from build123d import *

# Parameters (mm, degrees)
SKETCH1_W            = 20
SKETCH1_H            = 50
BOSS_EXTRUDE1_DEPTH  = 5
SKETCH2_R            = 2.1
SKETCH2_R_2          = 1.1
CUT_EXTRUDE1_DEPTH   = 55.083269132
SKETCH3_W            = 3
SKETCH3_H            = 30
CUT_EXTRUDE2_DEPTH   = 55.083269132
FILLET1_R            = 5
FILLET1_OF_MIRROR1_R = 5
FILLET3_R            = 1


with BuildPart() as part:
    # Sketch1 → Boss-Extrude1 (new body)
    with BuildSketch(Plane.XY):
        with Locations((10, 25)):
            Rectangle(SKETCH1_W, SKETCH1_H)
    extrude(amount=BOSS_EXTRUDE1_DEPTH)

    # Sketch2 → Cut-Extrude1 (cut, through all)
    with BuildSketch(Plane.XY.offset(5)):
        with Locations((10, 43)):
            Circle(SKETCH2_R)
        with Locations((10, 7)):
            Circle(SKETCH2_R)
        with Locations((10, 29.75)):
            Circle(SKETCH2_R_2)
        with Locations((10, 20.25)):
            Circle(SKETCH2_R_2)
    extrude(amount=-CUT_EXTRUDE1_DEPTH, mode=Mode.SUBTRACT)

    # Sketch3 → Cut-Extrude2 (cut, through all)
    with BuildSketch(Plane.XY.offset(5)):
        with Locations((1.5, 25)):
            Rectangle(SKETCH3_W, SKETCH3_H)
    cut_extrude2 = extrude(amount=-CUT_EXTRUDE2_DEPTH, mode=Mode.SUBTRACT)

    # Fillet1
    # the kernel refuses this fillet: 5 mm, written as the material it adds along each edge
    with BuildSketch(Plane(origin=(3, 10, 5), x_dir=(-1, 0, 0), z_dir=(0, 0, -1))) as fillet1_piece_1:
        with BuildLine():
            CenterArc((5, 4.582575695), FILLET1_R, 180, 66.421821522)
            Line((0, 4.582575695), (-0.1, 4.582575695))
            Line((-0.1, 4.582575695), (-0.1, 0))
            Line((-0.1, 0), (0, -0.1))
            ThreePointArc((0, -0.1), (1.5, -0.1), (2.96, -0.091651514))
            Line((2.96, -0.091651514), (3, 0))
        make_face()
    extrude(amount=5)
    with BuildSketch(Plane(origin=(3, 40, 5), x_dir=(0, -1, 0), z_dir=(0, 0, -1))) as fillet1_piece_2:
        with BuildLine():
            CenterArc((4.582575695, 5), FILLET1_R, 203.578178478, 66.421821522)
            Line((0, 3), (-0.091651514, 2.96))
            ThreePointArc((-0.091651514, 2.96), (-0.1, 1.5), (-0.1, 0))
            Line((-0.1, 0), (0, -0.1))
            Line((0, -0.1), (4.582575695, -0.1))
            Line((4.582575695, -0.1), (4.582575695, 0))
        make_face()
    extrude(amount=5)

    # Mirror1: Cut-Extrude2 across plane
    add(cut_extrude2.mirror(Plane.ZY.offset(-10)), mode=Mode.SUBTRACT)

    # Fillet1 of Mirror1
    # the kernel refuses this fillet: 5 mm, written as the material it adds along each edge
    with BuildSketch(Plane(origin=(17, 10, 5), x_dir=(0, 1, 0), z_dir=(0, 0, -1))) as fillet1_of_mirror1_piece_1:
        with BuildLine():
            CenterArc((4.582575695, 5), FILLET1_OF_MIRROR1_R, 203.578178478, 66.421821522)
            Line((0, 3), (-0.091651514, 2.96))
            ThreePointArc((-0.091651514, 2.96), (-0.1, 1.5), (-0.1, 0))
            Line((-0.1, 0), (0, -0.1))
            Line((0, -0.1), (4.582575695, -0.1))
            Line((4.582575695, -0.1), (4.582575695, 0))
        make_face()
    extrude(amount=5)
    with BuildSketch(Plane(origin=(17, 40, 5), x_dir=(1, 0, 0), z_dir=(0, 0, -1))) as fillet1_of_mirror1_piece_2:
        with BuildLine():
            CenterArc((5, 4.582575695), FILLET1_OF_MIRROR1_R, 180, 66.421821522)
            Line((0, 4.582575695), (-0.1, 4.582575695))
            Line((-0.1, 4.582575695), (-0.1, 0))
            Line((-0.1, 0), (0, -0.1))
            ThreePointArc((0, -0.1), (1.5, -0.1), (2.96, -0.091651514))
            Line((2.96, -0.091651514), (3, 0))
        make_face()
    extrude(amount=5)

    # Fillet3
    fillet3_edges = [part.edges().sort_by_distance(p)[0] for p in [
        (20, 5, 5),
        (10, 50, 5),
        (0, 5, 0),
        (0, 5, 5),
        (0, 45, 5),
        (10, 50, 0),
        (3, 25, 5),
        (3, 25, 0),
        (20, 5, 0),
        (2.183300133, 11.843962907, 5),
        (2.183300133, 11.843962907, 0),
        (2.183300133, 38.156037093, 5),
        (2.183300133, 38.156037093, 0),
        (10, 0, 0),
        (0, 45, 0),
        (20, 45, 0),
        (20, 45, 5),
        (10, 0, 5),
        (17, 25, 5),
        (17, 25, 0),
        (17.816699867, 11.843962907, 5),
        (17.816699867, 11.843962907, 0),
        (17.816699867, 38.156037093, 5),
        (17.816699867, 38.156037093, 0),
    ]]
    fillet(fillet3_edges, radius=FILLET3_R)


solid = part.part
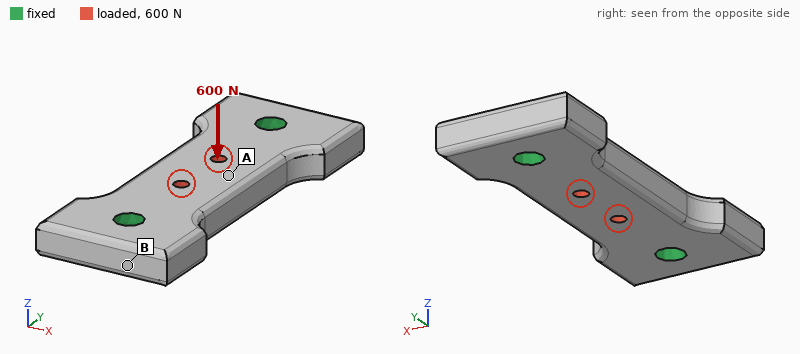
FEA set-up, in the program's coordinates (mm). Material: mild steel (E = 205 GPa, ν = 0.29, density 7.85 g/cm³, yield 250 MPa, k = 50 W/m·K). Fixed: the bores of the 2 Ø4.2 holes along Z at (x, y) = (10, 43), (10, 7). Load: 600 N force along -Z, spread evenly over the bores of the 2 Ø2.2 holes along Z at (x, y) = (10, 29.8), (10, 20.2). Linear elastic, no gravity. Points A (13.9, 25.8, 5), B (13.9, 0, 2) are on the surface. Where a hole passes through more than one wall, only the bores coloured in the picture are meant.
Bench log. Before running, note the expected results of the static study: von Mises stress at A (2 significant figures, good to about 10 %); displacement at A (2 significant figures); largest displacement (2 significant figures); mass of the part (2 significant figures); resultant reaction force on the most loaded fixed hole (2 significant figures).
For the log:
23 MPa
4.3 µm
4.4 µm
31 g
300 N
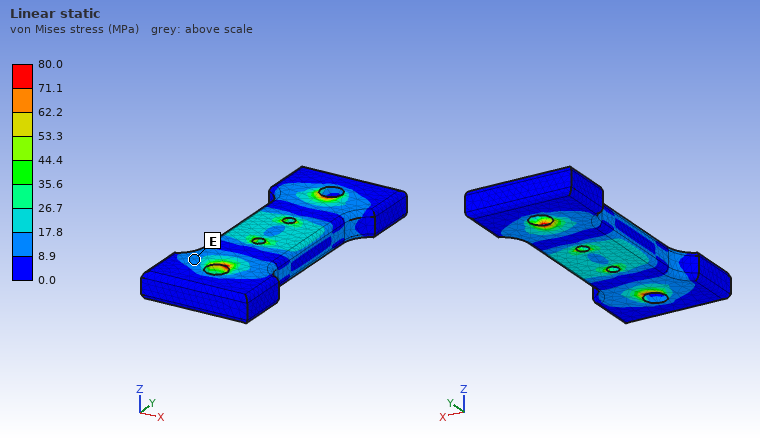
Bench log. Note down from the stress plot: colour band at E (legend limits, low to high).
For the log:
8.9 to 17.8 MPa
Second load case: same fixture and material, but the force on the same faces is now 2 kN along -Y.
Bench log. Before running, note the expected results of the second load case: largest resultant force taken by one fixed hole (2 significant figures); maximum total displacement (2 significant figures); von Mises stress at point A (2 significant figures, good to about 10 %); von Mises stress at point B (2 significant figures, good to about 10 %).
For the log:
1.0 kN
1.5 µm
10.0 MPa
4.2 MPa
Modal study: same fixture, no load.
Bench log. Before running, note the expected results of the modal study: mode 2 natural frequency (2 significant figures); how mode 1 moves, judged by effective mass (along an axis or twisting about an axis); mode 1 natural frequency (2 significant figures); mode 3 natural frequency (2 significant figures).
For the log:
27 kHz
along Z
19 kHz
28 kHz
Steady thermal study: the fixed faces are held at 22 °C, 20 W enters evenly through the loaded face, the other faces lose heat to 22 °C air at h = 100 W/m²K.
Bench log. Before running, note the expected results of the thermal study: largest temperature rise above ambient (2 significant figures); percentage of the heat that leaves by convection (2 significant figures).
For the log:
40 K
14 %
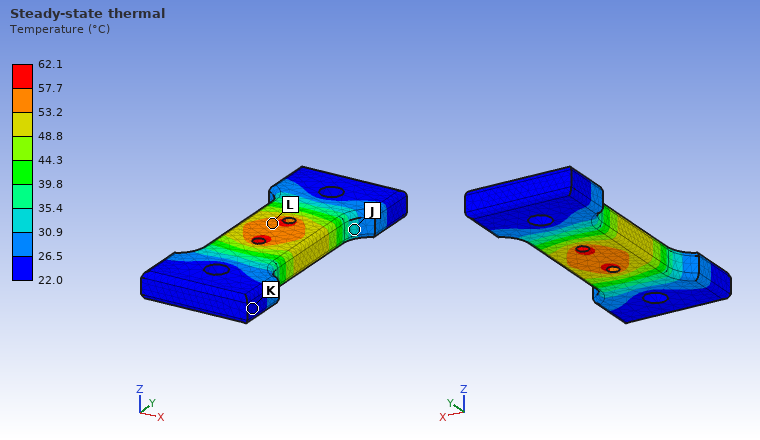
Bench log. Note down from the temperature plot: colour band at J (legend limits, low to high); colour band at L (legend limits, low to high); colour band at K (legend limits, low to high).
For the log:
30.9 to 35.4 °C
53.2 to 57.7 °C
22.0 to 26.5 °C
